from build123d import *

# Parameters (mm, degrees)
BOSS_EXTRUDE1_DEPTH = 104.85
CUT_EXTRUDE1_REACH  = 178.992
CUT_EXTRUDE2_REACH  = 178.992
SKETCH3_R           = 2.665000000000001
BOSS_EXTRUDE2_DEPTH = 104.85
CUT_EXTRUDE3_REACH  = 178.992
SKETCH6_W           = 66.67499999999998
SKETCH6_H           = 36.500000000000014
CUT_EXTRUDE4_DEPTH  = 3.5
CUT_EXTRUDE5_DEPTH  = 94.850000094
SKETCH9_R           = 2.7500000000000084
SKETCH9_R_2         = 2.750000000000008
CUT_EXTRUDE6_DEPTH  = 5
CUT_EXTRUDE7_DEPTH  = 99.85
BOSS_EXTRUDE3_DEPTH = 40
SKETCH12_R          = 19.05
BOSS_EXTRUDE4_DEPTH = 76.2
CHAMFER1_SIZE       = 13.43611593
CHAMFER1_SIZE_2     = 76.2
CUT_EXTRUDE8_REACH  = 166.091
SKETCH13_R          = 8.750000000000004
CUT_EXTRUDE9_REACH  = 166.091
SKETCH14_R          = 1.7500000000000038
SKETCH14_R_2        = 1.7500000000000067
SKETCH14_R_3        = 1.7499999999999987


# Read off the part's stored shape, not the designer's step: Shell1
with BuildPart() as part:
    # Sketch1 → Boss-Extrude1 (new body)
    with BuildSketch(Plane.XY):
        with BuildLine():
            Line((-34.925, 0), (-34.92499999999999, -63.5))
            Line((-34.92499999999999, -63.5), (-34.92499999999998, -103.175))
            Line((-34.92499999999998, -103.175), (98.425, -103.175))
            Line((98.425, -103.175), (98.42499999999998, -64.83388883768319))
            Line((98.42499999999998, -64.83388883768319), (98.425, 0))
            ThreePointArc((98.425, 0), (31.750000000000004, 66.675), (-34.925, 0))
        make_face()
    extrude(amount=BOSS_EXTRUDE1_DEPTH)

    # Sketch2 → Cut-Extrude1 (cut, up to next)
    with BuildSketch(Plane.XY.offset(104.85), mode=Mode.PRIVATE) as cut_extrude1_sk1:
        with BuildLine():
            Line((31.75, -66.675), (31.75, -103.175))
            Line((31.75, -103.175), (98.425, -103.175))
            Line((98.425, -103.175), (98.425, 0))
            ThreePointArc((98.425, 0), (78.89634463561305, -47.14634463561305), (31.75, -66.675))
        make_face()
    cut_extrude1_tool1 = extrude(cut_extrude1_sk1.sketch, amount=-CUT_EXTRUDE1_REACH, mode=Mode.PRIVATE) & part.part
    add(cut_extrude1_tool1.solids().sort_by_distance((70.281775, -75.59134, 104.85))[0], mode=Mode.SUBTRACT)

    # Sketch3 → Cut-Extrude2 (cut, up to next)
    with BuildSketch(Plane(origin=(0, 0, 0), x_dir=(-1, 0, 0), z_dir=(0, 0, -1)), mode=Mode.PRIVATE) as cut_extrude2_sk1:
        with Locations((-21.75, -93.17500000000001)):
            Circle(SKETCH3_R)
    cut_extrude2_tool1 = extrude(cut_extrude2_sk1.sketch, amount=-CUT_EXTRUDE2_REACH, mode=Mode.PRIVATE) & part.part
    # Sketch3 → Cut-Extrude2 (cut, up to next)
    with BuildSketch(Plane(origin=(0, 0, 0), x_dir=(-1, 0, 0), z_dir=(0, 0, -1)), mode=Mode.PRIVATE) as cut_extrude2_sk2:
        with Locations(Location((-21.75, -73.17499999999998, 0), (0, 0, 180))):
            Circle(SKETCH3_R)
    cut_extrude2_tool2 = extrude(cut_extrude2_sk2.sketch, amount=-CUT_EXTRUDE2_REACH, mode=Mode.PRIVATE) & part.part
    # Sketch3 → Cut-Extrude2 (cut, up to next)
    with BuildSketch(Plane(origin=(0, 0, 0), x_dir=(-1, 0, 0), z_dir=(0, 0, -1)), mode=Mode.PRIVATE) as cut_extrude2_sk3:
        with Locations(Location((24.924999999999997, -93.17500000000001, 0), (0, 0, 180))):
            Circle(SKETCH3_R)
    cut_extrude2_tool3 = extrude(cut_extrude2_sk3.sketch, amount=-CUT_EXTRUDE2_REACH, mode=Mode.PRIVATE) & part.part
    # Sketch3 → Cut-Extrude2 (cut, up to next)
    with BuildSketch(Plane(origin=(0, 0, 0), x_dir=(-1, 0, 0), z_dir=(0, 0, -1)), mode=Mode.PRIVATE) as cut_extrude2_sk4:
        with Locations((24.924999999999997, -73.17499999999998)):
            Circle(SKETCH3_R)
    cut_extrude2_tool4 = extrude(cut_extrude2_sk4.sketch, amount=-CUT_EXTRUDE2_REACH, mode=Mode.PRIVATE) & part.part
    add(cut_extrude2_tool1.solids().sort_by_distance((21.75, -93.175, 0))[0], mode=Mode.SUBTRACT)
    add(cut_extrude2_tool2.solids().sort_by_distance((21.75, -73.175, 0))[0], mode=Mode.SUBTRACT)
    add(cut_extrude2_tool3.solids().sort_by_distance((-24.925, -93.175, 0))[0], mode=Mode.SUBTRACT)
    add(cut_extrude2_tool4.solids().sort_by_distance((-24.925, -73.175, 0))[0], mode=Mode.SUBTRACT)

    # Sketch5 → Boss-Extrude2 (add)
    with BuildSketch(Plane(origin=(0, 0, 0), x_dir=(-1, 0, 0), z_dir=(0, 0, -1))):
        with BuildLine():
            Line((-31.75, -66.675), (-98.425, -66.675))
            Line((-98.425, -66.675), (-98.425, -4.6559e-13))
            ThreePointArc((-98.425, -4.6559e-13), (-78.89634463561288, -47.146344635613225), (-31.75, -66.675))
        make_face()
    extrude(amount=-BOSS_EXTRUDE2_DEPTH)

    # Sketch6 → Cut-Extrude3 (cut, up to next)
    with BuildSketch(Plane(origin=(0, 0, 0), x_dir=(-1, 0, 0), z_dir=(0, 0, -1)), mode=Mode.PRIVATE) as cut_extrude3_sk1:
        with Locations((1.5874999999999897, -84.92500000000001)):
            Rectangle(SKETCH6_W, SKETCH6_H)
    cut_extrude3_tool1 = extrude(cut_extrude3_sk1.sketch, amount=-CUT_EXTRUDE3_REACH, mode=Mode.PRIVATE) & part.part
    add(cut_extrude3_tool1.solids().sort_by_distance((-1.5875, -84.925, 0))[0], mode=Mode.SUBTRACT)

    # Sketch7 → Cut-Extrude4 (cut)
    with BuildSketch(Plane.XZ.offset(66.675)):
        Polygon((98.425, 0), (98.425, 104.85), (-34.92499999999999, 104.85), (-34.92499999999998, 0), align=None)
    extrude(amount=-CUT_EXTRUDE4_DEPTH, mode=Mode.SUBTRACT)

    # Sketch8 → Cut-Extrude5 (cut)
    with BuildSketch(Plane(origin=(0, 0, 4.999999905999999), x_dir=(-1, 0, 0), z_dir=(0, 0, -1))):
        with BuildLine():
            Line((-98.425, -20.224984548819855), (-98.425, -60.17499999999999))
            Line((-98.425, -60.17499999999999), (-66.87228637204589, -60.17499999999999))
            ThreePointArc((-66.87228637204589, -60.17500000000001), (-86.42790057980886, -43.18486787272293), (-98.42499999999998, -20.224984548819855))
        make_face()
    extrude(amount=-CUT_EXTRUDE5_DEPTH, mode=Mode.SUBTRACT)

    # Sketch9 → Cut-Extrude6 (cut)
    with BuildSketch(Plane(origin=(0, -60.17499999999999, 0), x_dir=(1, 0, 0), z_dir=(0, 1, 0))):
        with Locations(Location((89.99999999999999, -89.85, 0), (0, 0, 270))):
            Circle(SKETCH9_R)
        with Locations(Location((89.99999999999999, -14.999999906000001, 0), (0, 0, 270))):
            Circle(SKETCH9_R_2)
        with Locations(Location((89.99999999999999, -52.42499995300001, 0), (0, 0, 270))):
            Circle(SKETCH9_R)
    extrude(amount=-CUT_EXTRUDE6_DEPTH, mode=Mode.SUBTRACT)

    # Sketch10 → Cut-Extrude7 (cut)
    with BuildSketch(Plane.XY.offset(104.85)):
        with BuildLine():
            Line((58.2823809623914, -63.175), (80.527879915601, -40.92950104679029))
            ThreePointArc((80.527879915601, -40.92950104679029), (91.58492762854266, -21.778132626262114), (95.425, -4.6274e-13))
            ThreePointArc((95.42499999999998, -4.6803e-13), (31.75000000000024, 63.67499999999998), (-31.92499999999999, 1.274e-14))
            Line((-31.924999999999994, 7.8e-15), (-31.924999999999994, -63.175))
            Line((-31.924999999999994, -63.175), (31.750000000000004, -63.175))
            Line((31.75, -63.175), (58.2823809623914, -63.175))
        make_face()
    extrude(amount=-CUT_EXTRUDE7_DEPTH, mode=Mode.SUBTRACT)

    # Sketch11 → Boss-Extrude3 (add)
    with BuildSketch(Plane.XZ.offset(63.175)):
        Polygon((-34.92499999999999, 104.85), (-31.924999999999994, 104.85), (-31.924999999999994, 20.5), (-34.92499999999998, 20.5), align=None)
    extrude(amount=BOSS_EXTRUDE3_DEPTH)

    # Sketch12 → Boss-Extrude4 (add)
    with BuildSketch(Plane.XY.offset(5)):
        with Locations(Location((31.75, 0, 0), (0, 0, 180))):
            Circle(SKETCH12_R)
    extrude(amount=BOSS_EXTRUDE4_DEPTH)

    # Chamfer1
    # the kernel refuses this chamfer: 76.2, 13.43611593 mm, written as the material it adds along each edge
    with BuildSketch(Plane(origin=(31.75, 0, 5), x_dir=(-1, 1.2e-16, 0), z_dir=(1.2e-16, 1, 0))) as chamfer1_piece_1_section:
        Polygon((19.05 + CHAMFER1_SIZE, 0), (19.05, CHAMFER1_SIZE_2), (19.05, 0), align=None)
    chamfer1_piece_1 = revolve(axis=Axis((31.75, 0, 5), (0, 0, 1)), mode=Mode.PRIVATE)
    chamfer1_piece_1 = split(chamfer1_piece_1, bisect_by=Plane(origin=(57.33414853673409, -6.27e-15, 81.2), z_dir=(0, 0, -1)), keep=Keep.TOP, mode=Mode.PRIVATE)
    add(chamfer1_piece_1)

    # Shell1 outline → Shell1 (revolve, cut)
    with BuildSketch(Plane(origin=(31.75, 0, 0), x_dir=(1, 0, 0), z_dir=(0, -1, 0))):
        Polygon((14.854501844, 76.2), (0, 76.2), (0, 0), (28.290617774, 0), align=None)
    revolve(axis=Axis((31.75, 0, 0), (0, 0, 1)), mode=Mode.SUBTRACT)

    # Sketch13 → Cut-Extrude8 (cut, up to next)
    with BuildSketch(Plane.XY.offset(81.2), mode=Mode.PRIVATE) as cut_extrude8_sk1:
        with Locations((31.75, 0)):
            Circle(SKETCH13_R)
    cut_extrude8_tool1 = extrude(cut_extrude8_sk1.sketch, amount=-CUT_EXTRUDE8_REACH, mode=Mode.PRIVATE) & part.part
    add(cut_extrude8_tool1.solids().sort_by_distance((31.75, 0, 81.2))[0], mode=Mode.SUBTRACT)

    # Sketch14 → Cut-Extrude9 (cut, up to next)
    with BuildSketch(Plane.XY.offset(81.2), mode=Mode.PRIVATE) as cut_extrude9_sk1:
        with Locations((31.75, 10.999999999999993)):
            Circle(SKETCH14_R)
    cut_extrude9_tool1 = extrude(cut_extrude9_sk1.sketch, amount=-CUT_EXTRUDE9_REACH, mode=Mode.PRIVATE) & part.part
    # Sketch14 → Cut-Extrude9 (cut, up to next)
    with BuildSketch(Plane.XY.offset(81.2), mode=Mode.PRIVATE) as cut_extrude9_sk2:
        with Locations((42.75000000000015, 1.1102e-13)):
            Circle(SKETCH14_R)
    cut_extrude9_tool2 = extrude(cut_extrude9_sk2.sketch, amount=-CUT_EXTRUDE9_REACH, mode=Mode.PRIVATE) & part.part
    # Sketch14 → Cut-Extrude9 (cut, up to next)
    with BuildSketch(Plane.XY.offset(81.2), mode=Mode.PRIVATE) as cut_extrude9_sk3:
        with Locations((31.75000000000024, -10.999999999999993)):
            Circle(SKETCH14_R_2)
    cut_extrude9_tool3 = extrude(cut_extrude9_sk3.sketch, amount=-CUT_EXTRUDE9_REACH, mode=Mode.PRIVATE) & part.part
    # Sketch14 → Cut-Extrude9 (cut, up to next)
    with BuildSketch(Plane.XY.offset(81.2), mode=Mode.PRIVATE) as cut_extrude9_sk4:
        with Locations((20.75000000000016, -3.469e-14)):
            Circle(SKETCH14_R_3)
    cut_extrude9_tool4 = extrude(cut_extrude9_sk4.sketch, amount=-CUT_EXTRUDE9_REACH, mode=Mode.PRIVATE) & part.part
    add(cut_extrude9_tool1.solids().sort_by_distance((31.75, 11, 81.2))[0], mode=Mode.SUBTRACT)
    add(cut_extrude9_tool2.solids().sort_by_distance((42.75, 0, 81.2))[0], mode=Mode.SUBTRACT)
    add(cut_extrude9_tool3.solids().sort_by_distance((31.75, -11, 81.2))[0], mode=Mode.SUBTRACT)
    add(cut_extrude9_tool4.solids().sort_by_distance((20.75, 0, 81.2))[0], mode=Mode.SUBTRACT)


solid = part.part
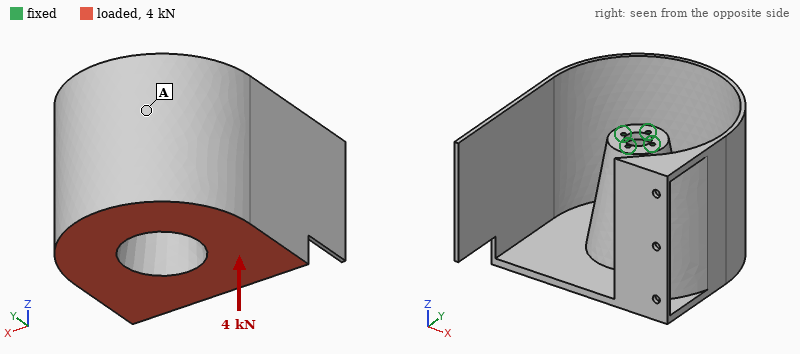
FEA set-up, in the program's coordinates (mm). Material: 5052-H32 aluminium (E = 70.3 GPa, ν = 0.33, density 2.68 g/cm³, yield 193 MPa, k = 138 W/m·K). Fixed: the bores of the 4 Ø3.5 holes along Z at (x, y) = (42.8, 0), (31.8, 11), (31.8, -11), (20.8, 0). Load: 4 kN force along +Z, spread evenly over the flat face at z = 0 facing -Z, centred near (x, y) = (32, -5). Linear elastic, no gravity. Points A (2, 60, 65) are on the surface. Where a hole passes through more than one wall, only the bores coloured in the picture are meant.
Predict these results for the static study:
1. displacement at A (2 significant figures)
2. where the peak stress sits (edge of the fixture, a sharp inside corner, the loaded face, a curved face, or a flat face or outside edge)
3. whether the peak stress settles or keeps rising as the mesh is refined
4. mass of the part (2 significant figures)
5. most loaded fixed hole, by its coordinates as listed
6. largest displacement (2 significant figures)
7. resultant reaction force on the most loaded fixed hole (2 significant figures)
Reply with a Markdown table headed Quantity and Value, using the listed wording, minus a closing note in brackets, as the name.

| Quantity | Value |
|---|---|
| displacement at A | 0.13 mm |
| where the peak stress sits | edge of the fixture |
| whether the peak stress settles or keeps rising as the mesh is refined | keeps rising |
| mass of the part | 710 g |
| most loaded fixed hole, by its coordinates as listed | (31.8, -11) |
| largest displacement | 0.49 mm |
| resultant reaction force on the most loaded fixed hole | 1.7 kN |
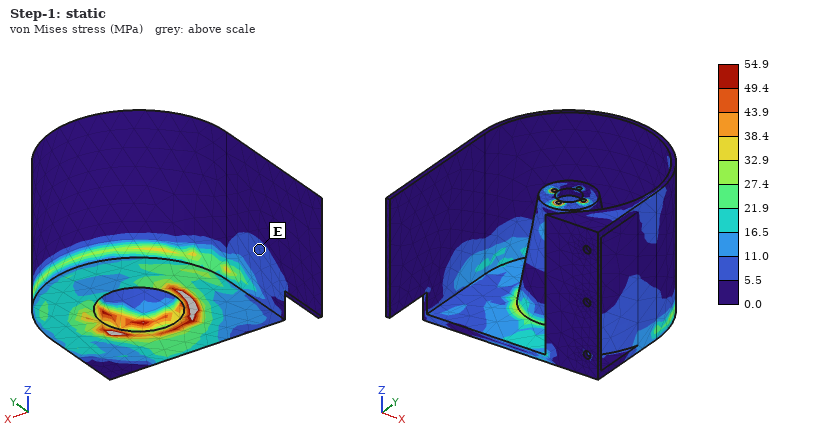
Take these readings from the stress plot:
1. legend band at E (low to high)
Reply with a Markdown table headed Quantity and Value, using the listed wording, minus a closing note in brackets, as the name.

| Quantity | Value |
|---|---|
| legend band at E | 5.5 to 11.0 MPa |
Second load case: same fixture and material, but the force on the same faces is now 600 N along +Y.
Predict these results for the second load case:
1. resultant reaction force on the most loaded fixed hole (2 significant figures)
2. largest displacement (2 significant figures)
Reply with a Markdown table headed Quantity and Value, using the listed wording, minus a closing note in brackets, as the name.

| Quantity | Value |
|---|---|
| resultant reaction force on the most loaded fixed hole | 1.5 kN |
| largest displacement | 0.11 mm |
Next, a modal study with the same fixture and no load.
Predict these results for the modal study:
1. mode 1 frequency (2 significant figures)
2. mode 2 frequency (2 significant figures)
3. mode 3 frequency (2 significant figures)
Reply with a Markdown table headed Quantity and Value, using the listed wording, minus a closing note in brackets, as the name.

| Quantity | Value |
|---|---|
| mode 1 frequency | 240 Hz |
| mode 2 frequency | 350 Hz |
| mode 3 frequency | 420 Hz |
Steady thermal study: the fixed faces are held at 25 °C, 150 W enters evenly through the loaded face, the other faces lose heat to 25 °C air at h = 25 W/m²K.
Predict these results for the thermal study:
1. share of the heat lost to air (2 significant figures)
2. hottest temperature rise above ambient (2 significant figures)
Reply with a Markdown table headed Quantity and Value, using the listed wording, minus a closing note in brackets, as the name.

| Quantity | Value |
|---|---|
| share of the heat lost to air | 68 % |
| hottest temperature rise above ambient | 56 K |
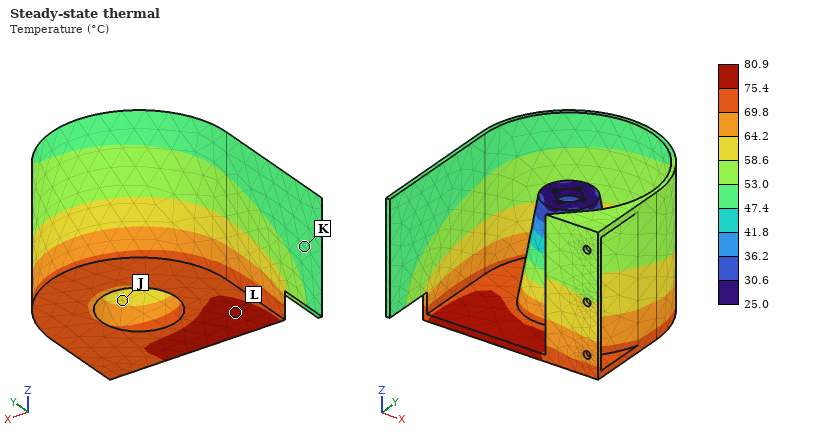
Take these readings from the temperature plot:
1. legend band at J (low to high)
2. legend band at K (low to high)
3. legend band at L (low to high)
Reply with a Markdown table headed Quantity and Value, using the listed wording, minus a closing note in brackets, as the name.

| Quantity | Value |
|---|---|
| legend band at J | 58.6 to 64.2 °C |
| legend band at K | 47.4 to 53.0 °C |
| legend band at L | 75.4 to 80.9 °C |
